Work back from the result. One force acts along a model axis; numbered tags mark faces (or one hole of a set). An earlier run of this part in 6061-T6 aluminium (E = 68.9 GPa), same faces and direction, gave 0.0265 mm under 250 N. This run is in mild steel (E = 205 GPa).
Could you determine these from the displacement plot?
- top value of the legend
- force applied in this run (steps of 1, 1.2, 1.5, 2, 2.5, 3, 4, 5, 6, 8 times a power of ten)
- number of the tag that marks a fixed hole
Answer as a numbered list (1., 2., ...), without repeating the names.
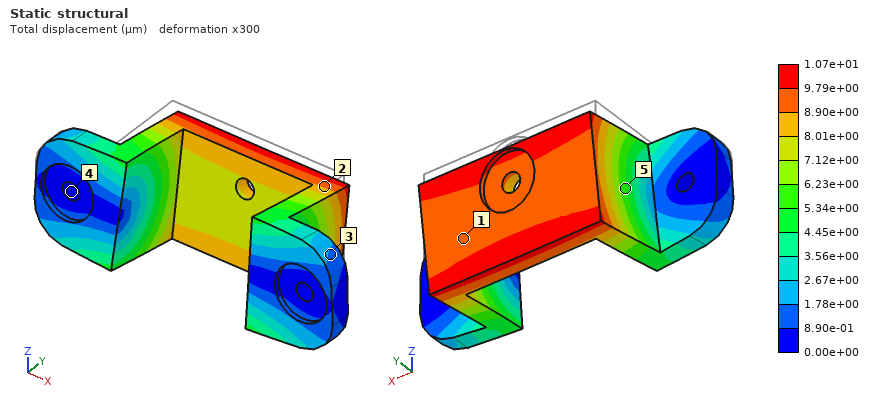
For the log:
1. 1.07e+01 µm
2. 300 N
3. 4
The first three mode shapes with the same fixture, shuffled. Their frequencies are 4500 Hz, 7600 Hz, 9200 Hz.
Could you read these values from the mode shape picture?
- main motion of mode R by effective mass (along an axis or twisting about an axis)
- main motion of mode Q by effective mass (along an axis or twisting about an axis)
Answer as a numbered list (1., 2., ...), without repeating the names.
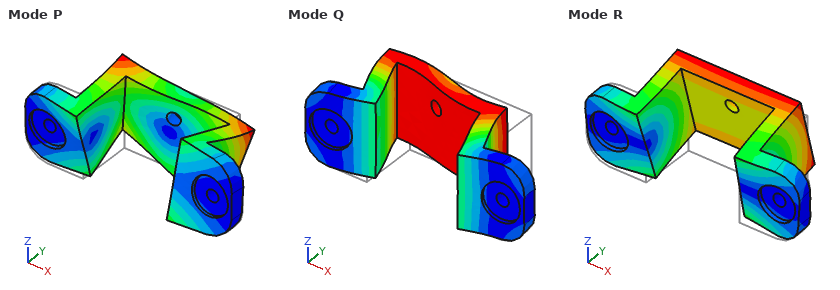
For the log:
1. along Z
2. along X
